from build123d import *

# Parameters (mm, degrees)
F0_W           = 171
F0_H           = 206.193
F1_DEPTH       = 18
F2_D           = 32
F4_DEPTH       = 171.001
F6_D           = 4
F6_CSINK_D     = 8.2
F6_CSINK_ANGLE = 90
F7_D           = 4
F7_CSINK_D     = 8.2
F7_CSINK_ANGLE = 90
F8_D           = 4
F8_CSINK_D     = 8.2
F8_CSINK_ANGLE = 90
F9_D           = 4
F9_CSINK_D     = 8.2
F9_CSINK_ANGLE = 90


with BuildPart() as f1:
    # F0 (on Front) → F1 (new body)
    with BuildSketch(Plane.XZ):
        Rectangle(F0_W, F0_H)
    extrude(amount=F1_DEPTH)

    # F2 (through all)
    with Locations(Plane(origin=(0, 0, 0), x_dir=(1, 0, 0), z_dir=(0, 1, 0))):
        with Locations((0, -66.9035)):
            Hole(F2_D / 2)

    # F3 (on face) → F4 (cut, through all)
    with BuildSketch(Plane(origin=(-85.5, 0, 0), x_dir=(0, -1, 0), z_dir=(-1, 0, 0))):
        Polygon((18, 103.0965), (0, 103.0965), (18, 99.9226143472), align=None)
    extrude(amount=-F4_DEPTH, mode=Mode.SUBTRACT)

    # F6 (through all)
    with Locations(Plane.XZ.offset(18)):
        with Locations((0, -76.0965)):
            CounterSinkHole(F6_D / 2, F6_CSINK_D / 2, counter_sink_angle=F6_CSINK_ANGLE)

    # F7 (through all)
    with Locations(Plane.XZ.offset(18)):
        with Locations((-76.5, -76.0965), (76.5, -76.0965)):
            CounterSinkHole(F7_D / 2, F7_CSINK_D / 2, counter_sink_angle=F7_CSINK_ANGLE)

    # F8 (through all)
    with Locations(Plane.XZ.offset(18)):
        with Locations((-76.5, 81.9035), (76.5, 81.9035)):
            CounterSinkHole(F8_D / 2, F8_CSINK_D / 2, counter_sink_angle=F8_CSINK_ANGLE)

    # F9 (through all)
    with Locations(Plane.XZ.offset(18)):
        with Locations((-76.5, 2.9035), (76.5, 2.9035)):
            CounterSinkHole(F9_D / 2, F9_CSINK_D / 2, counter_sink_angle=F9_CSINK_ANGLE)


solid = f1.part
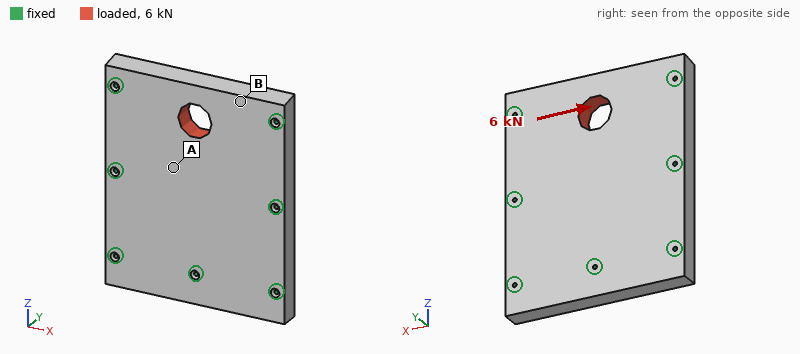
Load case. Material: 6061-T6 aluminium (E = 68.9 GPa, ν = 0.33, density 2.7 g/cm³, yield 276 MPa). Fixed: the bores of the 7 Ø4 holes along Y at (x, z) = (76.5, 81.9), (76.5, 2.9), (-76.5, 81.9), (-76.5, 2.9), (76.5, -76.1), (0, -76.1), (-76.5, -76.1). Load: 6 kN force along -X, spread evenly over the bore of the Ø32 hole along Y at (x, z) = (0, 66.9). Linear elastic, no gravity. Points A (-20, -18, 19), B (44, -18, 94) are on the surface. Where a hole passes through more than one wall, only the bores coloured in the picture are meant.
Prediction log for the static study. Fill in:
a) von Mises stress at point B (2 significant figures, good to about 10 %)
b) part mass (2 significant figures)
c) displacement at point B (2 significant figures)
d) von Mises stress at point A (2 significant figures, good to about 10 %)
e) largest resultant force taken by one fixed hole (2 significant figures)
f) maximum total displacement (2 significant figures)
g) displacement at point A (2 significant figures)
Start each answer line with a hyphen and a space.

- 2.2 MPa
- 1.7 kg
- 2.1 µm
- 1.1 MPa
- 1.9 kN
- 3.8 µm
- 1.3 µm
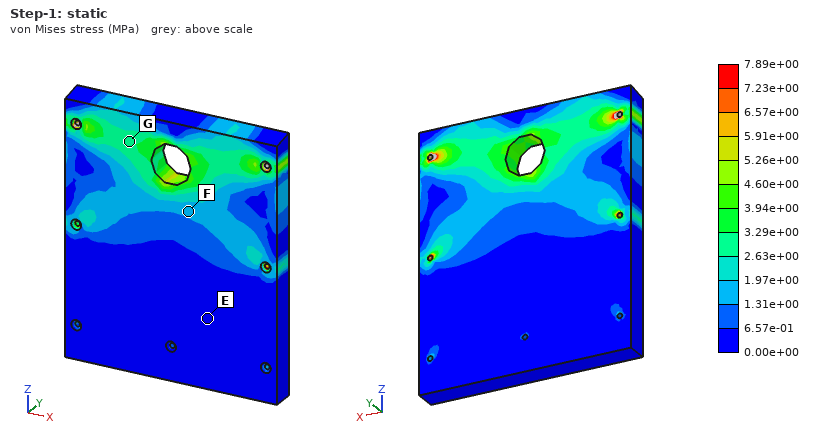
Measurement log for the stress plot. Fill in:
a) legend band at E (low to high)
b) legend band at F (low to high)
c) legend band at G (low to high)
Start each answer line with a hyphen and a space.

- 0.00e+00 to 6.57e-01 MPa
- 1.31e+00 to 1.97e+00 MPa
- 2.63e+00 to 3.29e+00 MPa
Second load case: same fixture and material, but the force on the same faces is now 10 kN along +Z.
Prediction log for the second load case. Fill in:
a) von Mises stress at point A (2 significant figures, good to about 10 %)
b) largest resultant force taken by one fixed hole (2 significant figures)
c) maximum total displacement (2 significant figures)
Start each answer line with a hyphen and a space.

- 4.0 MPa
- 2.2 kN
- 12 µm
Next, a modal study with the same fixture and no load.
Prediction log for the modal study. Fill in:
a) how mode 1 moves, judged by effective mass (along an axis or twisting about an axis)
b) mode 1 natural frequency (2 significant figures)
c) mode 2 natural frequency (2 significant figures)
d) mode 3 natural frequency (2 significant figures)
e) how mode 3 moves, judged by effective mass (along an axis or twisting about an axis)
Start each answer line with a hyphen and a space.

- along Y
- 2900 Hz
- 4500 Hz
- 7000 Hz
- twisting about Z
